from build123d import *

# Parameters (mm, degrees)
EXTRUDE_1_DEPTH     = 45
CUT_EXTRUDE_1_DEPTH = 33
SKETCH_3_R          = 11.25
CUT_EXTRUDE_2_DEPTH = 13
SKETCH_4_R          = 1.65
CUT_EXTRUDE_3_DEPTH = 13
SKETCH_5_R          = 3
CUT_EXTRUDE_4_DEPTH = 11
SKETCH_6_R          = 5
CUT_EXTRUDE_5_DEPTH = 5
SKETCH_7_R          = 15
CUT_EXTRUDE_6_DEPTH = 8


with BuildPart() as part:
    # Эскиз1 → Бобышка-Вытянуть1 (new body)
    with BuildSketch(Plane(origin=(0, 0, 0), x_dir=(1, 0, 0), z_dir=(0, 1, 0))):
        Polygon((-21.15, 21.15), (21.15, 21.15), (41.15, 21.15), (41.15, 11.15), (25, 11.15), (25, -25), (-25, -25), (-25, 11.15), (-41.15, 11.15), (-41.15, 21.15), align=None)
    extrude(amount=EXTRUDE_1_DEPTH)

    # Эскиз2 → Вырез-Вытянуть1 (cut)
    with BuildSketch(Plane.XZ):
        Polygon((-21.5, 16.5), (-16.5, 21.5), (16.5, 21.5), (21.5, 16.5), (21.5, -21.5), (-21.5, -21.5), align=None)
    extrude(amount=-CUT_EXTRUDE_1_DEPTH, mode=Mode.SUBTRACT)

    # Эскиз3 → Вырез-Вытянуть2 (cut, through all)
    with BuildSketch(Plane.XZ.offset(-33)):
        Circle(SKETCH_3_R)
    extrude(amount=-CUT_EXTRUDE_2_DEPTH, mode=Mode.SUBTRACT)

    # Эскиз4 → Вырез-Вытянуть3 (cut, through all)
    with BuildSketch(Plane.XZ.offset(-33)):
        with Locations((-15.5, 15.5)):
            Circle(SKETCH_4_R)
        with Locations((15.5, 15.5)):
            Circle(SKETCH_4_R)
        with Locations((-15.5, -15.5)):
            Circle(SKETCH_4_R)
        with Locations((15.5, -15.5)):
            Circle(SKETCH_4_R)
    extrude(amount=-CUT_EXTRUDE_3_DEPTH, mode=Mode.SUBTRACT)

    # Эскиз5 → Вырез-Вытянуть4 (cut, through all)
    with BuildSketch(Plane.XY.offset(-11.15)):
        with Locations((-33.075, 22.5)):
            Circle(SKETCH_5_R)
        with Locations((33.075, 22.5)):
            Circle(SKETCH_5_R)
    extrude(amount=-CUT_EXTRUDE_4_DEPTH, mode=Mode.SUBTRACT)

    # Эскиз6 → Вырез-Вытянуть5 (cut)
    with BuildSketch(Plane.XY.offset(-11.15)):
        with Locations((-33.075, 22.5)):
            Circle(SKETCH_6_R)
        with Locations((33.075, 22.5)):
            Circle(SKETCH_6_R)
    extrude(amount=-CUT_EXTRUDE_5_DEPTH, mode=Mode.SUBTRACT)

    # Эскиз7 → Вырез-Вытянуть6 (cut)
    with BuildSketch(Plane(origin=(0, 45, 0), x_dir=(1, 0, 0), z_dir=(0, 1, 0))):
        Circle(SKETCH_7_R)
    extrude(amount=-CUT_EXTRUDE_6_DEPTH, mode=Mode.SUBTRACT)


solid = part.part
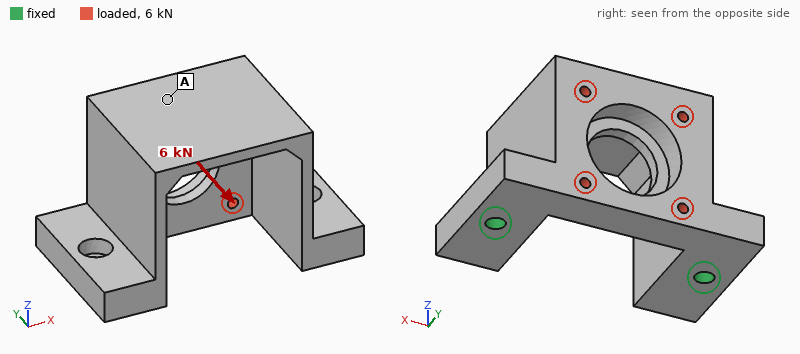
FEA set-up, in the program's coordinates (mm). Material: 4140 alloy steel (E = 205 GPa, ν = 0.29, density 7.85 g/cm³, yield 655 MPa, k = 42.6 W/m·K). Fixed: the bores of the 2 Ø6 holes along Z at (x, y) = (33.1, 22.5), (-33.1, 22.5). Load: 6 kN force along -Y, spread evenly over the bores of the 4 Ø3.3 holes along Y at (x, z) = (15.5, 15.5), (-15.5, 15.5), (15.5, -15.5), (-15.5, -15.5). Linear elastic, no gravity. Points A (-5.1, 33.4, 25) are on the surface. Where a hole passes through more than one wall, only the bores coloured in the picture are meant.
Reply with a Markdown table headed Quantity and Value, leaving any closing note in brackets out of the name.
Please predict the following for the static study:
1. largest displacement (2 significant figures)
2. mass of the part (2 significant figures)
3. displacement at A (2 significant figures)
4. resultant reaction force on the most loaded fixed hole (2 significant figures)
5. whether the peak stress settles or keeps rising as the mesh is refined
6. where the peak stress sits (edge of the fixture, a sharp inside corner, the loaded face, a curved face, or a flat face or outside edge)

| Quantity | Value |
|---|---|
| largest displacement | 0.13 mm |
| mass of the part | 390 g |
| displacement at A | 0.12 mm |
| resultant reaction force on the most loaded fixed hole | 3.4 kN |
| whether the peak stress settles or keeps rising as the mesh is refined | keeps rising |
| where the peak stress sits | edge of the fixture |
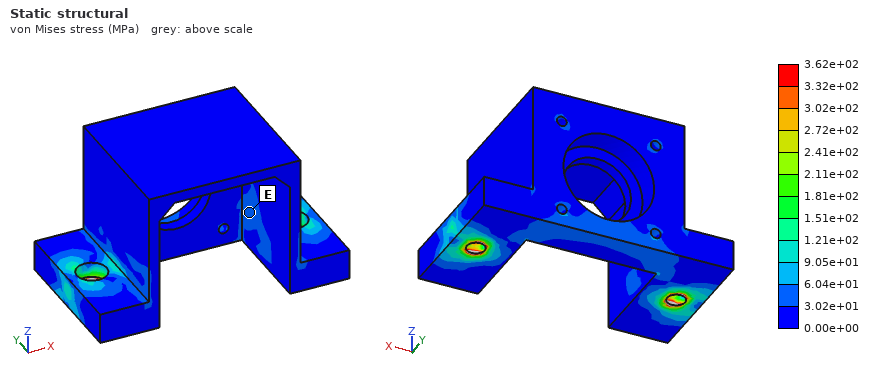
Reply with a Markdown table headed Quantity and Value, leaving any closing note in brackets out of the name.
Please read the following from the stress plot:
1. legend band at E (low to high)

| Quantity | Value |
|---|---|
| legend band at E | 3.02e+01 to 6.04e+01 MPa |
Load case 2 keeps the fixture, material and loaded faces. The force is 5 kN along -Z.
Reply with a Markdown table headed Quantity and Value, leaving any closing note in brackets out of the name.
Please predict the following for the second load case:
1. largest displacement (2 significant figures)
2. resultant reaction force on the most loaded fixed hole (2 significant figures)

| Quantity | Value |
|---|---|
| largest displacement | 91 µm |
| resultant reaction force on the most loaded fixed hole | 2.5 kN |
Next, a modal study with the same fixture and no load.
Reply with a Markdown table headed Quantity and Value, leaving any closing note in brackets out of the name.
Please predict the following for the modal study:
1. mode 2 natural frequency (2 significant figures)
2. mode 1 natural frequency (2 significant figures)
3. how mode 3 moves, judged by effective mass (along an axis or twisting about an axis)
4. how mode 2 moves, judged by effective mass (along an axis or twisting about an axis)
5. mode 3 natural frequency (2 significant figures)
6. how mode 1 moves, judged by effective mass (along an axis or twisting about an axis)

| Quantity | Value |
|---|---|
| mode 2 natural frequency | 3000 Hz |
| mode 1 natural frequency | 1900 Hz |
| how mode 3 moves, judged by effective mass | along X |
| how mode 2 moves, judged by effective mass | along X |
| mode 3 natural frequency | 6700 Hz |
| how mode 1 moves, judged by effective mass | along Y |
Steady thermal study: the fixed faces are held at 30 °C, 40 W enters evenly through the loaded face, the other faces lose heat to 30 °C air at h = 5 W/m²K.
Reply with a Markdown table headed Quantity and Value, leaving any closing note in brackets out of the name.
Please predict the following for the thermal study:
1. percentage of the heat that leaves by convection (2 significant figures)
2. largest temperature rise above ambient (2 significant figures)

| Quantity | Value |
|---|---|
| percentage of the heat that leaves by convection | 9.6 % |
| largest temperature rise above ambient | 65 K |
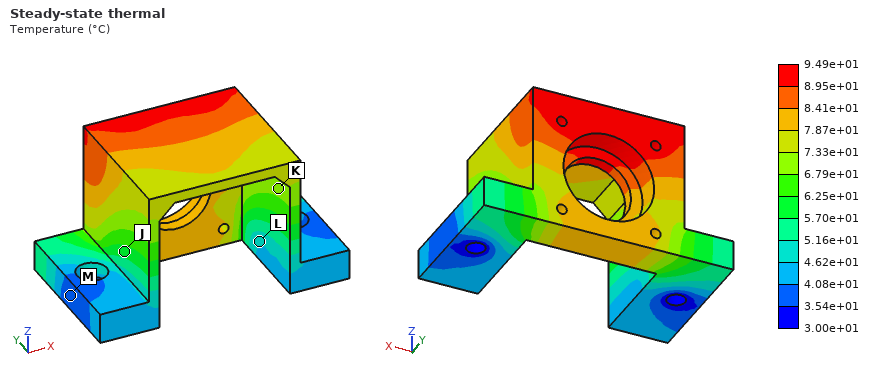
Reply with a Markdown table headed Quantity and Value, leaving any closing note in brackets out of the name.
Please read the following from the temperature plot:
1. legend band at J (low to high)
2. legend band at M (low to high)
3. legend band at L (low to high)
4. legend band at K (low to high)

| Quantity | Value |
|---|---|
| legend band at J | 5.70e+01 to 6.25e+01 °C |
| legend band at M | 3.54e+01 to 4.08e+01 °C |
| legend band at L | 4.62e+01 to 5.16e+01 °C |
| legend band at K | 6.79e+01 to 7.33e+01 °C |
